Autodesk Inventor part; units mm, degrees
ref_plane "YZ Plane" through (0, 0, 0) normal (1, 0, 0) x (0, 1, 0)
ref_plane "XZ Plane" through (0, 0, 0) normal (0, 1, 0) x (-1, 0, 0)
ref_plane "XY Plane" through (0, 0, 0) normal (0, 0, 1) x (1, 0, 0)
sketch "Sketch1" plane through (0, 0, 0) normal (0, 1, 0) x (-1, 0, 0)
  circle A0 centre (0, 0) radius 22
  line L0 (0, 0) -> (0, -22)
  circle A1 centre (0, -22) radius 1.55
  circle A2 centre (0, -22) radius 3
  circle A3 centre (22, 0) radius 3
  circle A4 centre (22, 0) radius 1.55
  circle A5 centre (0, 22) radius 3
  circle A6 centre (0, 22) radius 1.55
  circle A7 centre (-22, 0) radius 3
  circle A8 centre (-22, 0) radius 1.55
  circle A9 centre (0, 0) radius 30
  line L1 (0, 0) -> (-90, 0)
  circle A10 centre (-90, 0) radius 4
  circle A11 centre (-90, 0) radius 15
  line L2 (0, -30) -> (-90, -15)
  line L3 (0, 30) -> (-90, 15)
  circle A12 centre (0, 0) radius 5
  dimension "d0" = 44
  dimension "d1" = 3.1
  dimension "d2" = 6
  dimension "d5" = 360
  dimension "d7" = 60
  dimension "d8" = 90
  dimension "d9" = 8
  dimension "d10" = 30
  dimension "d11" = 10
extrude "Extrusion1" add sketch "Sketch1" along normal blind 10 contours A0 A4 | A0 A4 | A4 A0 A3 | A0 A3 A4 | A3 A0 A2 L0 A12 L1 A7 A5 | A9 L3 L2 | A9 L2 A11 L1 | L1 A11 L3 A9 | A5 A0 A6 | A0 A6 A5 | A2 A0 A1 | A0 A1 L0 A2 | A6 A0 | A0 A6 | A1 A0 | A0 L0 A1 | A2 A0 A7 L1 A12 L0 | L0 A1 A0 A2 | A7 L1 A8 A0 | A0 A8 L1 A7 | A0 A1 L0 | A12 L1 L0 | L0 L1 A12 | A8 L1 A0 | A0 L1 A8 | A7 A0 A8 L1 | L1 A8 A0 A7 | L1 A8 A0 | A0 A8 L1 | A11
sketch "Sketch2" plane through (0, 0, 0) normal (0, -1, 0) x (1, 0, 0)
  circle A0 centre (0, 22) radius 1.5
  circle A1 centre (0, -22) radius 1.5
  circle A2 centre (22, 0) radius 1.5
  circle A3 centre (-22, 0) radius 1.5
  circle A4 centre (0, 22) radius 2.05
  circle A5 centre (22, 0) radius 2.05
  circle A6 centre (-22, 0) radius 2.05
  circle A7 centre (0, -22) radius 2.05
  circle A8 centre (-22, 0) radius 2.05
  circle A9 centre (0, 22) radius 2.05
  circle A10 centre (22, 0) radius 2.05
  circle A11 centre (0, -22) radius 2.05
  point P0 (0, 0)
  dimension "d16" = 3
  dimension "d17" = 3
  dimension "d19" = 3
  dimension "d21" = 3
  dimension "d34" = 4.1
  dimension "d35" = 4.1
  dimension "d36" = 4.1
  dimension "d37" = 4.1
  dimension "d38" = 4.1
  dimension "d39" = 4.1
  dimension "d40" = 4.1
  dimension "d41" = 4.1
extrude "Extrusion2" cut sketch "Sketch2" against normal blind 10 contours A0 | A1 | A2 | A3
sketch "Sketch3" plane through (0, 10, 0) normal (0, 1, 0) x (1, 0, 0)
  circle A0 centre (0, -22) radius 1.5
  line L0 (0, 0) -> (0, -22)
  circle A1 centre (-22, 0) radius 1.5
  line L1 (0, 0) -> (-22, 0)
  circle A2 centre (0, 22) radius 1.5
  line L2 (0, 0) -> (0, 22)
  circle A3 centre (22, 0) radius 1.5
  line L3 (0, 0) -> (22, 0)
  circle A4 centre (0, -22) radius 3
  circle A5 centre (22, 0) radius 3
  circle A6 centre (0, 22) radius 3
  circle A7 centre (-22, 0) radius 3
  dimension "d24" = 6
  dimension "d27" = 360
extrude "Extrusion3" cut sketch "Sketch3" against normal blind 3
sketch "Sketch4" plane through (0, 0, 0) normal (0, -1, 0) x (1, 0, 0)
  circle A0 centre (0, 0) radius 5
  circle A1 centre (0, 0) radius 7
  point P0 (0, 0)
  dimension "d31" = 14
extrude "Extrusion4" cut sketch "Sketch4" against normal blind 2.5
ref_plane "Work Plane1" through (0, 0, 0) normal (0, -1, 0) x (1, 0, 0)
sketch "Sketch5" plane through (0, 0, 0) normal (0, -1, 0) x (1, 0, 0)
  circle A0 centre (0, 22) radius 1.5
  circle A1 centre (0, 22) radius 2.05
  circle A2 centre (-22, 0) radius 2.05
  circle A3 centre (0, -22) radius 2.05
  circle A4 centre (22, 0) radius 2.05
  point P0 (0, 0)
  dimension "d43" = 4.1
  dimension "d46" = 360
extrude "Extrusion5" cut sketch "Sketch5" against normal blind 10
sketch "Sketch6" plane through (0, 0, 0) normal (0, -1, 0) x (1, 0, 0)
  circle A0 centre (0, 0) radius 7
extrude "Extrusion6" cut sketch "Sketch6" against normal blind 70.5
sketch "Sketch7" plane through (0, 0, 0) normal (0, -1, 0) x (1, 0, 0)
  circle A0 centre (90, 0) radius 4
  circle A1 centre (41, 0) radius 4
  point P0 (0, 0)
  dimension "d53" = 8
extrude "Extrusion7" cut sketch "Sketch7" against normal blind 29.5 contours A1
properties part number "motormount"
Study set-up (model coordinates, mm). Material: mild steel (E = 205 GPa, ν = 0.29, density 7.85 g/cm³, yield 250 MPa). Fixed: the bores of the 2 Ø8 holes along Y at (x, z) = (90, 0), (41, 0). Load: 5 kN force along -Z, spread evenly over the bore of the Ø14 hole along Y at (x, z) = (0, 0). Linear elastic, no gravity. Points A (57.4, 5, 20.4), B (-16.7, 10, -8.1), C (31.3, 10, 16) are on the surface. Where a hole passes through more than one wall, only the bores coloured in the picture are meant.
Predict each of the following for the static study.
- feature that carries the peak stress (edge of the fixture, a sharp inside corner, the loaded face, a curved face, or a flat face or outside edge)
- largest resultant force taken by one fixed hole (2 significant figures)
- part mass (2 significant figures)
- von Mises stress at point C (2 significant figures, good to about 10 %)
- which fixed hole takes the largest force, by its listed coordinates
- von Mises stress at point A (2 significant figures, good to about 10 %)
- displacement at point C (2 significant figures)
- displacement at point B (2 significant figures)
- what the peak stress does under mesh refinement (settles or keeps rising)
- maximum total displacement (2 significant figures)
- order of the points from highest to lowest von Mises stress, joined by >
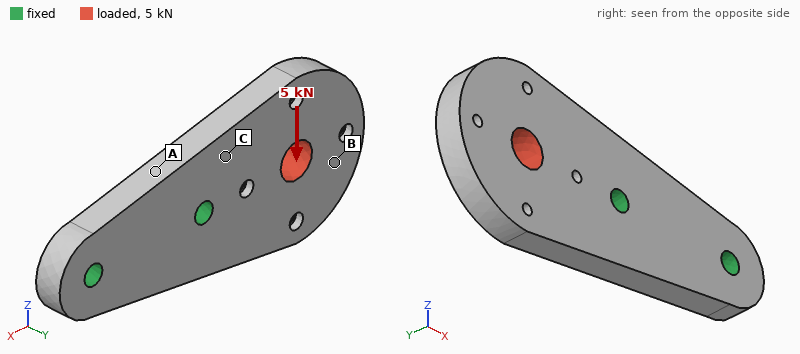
edge of the fixture
8.2 kN
430 g
29 MPa
(41, 0)
42 MPa
8.5 µm
36 µm
keeps rising
43 µm
A > C > B
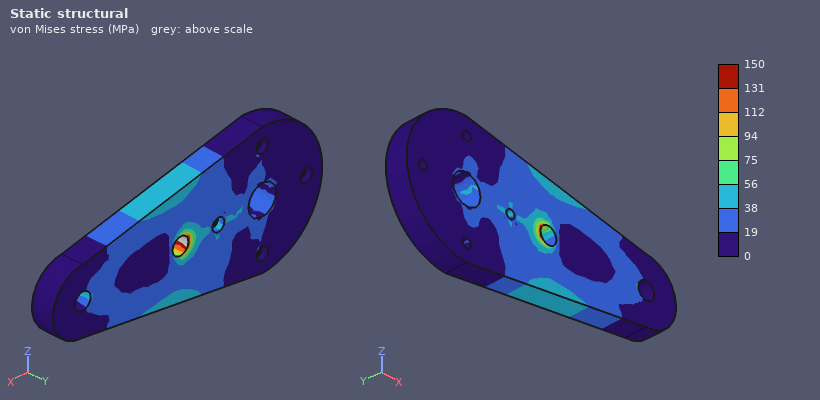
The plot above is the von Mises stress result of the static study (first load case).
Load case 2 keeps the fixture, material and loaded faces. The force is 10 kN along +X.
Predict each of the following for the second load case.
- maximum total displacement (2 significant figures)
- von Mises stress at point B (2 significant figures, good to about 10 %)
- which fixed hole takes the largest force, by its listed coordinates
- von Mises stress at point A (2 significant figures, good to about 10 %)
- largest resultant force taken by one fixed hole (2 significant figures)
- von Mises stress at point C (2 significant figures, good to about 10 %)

7.9 µm
9.9 MPa
(41, 0)
11 MPa
8.4 kN
16 MPa
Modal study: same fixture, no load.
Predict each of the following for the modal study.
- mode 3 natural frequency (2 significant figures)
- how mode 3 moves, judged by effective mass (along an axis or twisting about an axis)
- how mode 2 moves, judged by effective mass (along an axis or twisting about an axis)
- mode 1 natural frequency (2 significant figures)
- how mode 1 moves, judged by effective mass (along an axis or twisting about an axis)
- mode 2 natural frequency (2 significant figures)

4300 Hz
along Z
twisting about X
1700 Hz
along Y
3900 Hz
